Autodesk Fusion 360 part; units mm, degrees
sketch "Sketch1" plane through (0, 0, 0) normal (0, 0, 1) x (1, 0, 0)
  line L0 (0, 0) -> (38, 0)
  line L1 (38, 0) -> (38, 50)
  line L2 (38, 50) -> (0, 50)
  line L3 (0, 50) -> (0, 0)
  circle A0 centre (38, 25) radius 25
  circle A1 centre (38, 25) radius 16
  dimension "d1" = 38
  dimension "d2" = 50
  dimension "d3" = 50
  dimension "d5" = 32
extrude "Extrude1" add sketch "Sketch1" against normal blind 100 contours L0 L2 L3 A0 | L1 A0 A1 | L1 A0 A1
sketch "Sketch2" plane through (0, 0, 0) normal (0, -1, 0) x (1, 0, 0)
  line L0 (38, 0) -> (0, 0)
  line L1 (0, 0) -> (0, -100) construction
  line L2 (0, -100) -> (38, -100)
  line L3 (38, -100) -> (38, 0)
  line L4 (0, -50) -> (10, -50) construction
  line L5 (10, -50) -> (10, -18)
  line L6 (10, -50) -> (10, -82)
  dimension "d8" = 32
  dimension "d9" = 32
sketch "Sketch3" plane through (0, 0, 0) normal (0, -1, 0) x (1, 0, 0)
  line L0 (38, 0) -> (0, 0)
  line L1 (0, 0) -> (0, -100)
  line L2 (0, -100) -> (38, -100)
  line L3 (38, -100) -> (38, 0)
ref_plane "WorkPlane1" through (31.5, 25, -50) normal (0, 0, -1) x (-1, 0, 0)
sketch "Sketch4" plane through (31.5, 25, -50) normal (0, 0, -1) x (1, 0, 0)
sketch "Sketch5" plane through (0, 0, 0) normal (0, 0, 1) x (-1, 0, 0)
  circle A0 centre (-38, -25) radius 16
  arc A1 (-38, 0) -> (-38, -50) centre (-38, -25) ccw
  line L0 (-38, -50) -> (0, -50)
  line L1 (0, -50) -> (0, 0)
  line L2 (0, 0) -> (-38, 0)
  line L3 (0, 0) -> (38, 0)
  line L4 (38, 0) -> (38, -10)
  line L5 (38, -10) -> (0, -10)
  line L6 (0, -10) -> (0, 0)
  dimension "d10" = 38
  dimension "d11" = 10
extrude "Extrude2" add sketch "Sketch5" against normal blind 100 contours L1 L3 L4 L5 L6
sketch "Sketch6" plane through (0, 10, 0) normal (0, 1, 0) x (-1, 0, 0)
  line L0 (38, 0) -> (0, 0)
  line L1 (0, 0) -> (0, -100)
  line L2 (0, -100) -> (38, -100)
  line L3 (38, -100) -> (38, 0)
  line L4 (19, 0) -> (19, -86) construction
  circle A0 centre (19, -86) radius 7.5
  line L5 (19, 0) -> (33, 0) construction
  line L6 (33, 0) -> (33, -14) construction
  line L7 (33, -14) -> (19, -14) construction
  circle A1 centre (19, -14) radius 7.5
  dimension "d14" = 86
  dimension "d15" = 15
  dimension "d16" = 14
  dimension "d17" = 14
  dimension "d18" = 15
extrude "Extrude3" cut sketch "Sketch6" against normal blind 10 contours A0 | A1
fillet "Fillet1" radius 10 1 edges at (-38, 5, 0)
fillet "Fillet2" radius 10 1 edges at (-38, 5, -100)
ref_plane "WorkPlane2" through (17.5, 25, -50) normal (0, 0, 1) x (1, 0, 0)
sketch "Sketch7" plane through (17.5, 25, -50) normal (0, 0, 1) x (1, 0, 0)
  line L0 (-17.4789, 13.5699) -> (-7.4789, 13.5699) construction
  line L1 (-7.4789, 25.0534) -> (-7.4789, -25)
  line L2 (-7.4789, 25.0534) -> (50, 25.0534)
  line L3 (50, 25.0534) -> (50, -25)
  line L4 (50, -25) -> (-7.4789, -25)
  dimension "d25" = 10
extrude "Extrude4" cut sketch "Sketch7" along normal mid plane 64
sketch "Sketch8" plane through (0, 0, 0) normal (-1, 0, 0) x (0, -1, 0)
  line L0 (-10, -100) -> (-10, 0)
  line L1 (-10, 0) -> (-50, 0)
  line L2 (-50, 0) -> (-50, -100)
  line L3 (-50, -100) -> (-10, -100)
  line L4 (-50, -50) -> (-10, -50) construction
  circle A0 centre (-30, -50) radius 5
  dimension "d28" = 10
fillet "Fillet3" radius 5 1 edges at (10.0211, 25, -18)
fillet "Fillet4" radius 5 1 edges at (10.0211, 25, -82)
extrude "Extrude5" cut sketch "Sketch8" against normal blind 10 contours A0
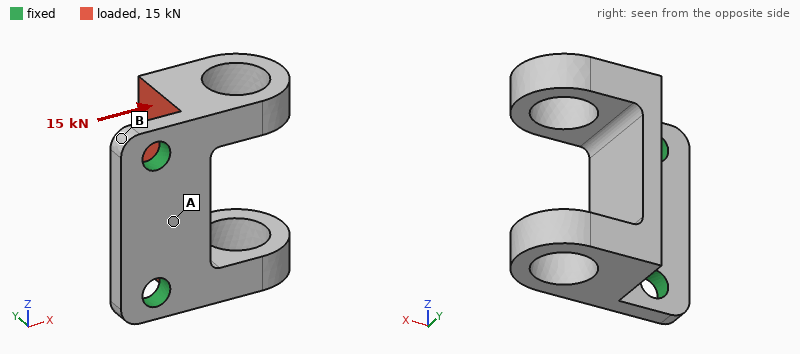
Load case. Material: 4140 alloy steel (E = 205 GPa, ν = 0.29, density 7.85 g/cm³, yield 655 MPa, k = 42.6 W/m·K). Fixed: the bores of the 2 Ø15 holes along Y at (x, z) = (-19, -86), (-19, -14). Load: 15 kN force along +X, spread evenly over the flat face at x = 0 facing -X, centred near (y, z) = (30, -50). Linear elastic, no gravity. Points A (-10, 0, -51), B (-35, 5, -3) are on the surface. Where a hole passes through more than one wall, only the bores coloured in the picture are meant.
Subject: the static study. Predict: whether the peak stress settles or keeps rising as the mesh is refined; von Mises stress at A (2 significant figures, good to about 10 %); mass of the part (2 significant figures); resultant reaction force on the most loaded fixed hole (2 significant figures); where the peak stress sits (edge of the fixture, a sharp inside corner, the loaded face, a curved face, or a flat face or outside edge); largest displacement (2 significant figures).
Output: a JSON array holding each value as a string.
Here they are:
["keeps rising", "110 MPa", "1.1 kg", "7.6 kN", "edge of the fixture", "0.37 mm"]
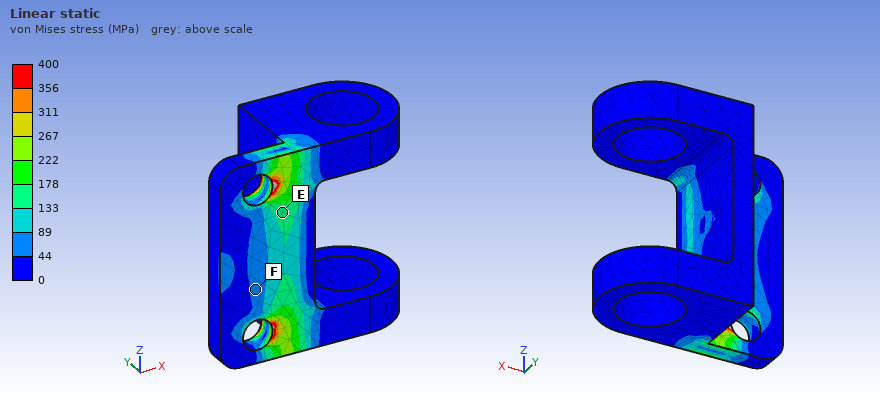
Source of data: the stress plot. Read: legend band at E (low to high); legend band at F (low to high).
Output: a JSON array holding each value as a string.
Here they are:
["133 to 178 MPa", "44 to 89 MPa"]
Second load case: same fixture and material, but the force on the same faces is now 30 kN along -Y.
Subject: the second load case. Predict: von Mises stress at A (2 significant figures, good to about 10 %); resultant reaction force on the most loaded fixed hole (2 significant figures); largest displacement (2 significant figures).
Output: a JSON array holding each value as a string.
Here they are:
["51 MPa", "15 kN", "0.16 mm"]
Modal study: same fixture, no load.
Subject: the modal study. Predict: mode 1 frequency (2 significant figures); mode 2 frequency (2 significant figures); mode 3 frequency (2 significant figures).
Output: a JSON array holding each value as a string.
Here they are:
["1200 Hz", "1700 Hz", "3100 Hz"]
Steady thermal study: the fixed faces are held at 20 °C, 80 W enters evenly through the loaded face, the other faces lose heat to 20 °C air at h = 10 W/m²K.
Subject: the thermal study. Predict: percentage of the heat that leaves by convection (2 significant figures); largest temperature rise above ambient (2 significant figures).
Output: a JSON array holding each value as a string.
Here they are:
["14 %", "72 K"]
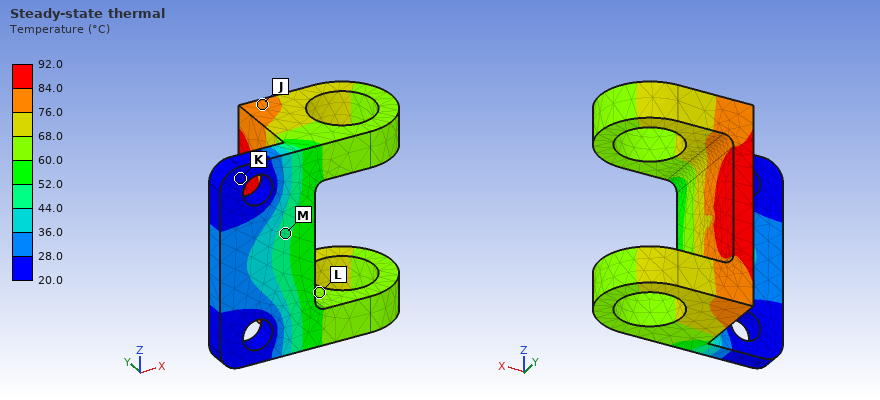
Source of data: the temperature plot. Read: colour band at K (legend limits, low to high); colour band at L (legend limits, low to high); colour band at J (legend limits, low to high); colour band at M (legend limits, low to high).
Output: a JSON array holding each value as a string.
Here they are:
["20.0 to 28.0 °C", "60.0 to 68.0 °C", "76.0 to 84.0 °C", "44.0 to 52.0 °C"]
